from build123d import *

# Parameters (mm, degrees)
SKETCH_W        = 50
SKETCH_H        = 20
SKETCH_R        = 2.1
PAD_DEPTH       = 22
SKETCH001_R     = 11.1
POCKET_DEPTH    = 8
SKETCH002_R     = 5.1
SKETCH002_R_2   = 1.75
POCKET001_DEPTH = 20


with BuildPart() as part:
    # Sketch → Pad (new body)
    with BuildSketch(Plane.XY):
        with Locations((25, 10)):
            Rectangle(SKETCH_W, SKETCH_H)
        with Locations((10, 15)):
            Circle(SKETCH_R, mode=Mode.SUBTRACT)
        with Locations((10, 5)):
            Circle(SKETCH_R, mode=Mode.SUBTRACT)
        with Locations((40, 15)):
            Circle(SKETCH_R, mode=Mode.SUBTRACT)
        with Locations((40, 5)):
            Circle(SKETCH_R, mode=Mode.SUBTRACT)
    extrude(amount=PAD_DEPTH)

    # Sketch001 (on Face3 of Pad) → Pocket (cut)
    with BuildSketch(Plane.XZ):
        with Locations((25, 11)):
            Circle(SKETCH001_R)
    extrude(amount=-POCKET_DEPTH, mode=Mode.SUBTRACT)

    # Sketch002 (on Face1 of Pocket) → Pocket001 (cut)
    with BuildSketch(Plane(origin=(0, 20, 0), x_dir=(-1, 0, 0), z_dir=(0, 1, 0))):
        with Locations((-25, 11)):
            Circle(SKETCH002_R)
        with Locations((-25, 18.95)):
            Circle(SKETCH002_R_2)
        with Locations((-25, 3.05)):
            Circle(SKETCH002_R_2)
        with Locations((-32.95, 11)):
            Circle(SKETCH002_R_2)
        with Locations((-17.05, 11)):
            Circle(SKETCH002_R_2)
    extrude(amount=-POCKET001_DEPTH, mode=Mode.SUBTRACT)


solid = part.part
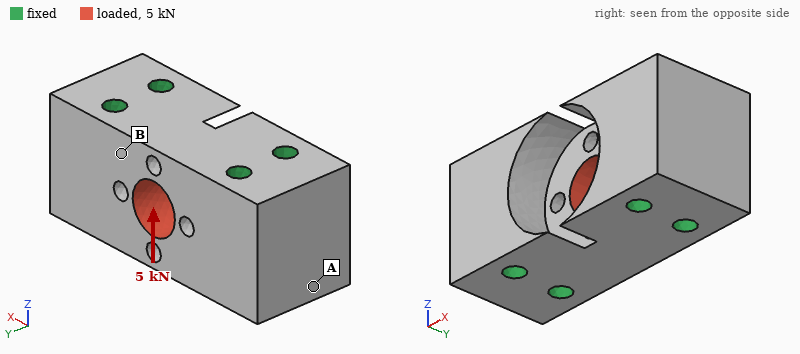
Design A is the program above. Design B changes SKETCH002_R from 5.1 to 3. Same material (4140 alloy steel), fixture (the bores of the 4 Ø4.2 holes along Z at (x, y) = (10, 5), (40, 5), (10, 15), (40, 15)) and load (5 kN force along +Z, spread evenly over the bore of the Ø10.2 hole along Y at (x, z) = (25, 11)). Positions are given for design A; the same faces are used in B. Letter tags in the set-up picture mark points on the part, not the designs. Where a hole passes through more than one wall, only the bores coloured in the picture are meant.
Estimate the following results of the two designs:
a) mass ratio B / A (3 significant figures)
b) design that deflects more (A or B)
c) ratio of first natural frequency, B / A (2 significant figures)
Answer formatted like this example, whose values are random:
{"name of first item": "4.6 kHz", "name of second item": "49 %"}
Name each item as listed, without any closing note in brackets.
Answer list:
{"mass ratio B / A": "1.04", "design that deflects more": "A", "ratio of first natural frequency, B / A": "0.93"}
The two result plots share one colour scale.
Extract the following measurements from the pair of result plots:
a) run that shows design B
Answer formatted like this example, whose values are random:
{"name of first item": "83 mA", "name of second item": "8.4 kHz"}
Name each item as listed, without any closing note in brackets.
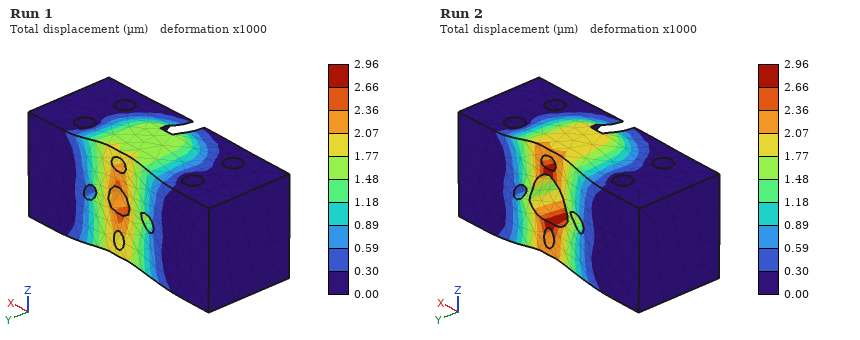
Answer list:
{"run that shows design B": "Run 1"}
